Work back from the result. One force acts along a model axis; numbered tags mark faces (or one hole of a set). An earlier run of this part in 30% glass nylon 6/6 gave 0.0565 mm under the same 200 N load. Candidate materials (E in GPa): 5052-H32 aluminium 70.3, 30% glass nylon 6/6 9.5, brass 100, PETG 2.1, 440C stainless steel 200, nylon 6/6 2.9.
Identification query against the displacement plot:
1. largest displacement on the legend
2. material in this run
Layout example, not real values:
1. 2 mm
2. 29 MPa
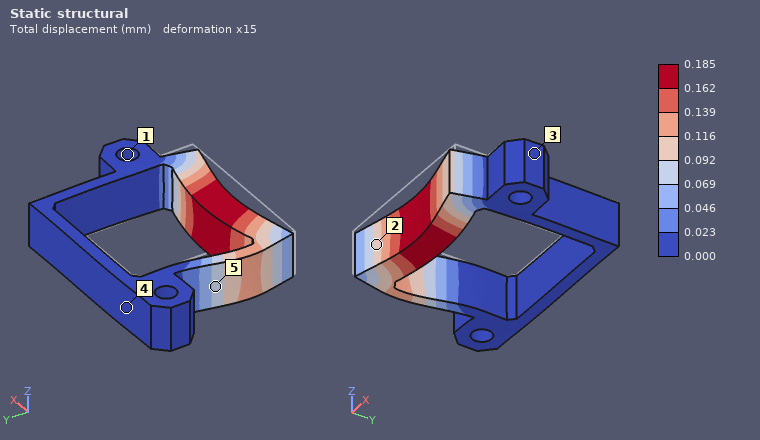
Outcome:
1. 0.185 mm
2. nylon 6/6
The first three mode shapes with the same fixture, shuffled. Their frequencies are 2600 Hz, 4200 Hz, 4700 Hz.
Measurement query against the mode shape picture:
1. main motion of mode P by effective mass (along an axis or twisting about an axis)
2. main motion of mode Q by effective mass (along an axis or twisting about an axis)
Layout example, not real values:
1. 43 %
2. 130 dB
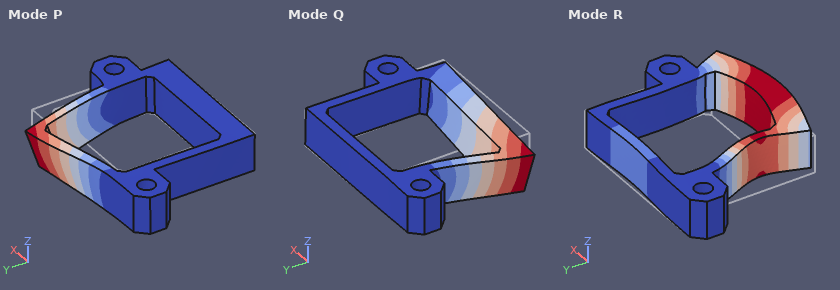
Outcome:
1. along Z
2. along Z
